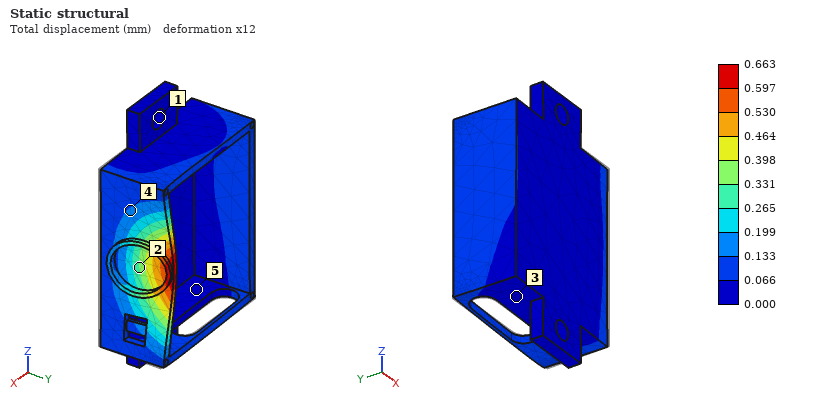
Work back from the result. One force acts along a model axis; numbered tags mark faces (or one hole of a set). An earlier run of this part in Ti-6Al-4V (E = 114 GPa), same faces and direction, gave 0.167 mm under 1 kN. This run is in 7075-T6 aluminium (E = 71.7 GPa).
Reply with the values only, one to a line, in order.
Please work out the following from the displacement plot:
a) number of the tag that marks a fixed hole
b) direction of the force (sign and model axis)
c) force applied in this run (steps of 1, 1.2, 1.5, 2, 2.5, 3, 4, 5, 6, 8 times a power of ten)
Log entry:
1
-X
2.5 kN
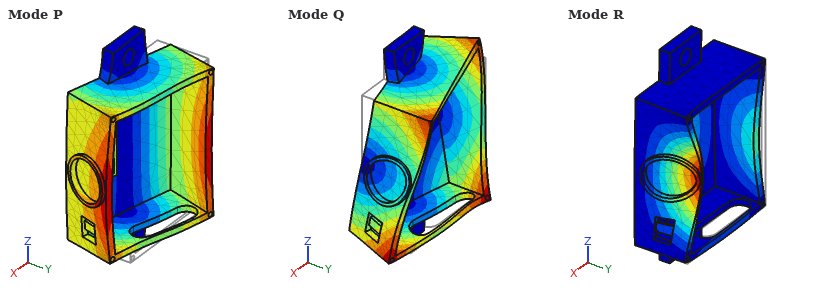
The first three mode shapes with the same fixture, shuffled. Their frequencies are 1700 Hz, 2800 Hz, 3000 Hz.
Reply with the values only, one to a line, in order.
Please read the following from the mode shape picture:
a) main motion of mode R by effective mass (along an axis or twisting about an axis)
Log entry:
along Y
